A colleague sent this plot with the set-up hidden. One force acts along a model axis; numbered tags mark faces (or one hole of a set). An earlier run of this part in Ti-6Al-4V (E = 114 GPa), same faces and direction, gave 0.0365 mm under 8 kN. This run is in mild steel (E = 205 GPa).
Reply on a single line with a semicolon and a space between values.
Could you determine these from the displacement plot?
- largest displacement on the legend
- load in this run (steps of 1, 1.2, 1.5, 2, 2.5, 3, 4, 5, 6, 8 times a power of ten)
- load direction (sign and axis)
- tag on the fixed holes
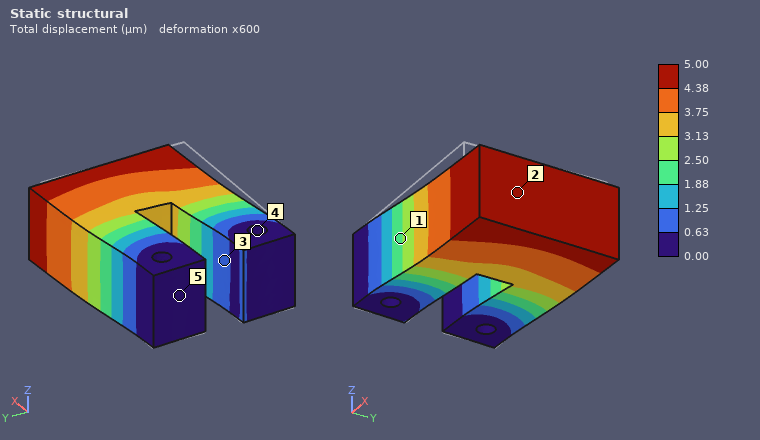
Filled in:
5.00 µm; 2 kN; +Y; 4
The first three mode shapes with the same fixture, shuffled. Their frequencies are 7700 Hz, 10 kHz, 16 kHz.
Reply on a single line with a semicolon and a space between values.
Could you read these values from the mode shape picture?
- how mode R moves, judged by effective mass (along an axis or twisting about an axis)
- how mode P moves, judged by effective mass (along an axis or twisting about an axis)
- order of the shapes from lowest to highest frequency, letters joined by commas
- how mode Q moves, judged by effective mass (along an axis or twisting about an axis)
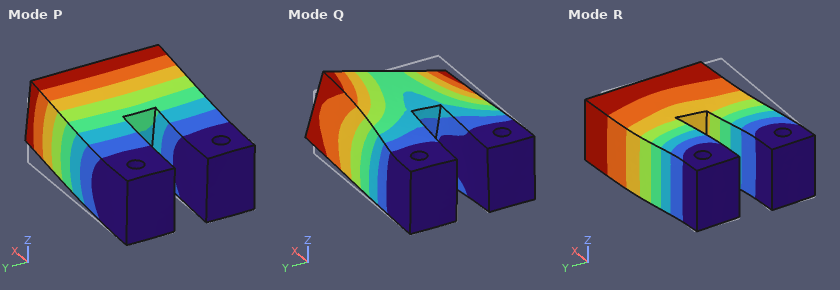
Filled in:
along Y; along Z; P, R, Q; twisting about X
